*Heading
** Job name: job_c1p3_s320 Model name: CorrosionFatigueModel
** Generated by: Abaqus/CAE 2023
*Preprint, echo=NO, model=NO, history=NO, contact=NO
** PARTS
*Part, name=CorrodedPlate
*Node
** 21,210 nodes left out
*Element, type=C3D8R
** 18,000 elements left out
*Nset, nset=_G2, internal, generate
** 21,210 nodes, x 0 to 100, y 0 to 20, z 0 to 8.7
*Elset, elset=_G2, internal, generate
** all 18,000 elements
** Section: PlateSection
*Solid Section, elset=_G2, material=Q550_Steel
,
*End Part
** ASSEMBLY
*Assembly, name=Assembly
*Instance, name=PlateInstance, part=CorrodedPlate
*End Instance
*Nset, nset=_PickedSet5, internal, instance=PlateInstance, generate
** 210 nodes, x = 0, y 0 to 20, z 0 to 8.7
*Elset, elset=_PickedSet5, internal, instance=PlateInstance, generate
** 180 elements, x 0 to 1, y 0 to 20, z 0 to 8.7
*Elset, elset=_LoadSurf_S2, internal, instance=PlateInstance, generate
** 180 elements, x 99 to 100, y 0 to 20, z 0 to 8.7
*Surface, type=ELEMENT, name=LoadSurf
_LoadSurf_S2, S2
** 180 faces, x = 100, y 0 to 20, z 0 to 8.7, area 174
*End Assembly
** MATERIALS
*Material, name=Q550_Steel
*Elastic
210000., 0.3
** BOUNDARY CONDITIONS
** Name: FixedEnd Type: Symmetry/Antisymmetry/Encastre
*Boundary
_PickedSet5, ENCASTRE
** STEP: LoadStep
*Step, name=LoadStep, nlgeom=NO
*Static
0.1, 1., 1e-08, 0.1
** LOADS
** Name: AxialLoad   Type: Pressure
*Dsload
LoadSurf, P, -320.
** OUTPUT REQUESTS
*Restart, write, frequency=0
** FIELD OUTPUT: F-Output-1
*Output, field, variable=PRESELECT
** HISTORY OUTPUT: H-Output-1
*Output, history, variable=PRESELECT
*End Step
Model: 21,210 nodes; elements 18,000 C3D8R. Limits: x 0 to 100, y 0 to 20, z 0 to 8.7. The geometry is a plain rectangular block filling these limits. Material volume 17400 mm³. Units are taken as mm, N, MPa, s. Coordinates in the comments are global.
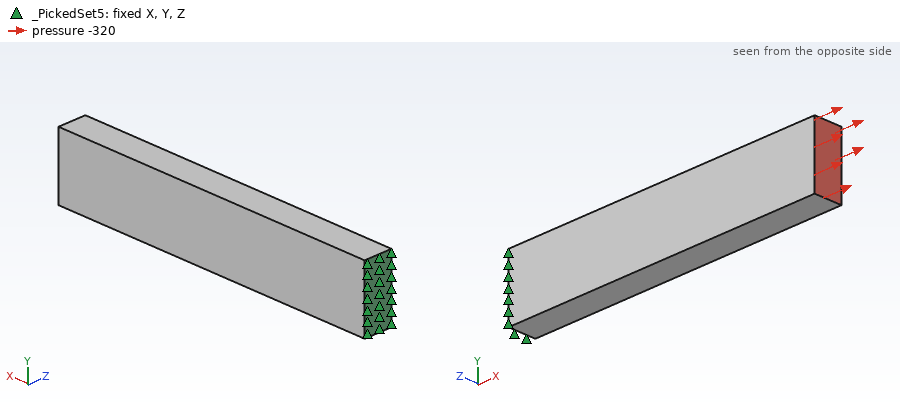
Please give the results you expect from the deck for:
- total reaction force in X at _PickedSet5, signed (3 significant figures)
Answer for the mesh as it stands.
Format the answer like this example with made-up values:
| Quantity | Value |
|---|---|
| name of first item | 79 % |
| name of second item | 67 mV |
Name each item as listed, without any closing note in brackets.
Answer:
| Quantity | Value |
|---|---|
| total reaction force in X at _PickedSet5, signed | -55700 N |
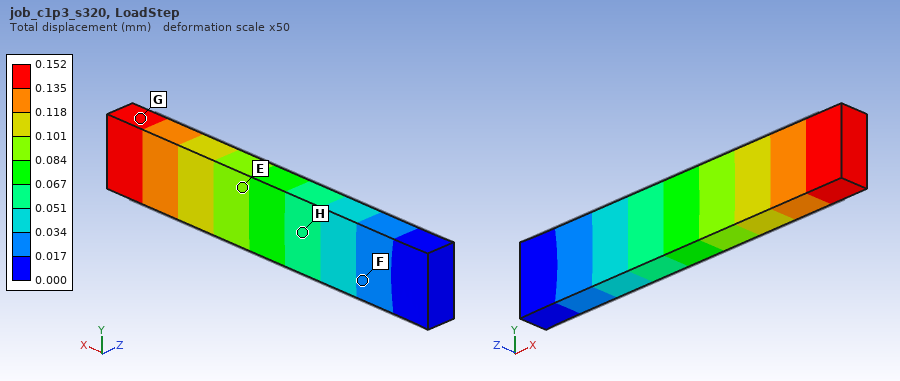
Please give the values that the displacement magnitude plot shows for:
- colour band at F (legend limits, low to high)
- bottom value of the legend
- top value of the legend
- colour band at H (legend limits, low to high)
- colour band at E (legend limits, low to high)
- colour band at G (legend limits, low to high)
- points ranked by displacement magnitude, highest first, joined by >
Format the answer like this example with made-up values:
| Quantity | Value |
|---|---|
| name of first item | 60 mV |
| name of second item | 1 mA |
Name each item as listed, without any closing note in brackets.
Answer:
| Quantity | Value |
|---|---|
| colour band at F | 0.017 to 0.034 mm |
| bottom value of the legend | 0.000 mm |
| top value of the legend | 0.152 mm |
| colour band at H | 0.051 to 0.067 mm |
| colour band at E | 0.084 to 0.101 mm |
| colour band at G | 0.135 to 0.152 mm |
| points ranked by displacement magnitude, highest first, joined by > | G > E > H > F |
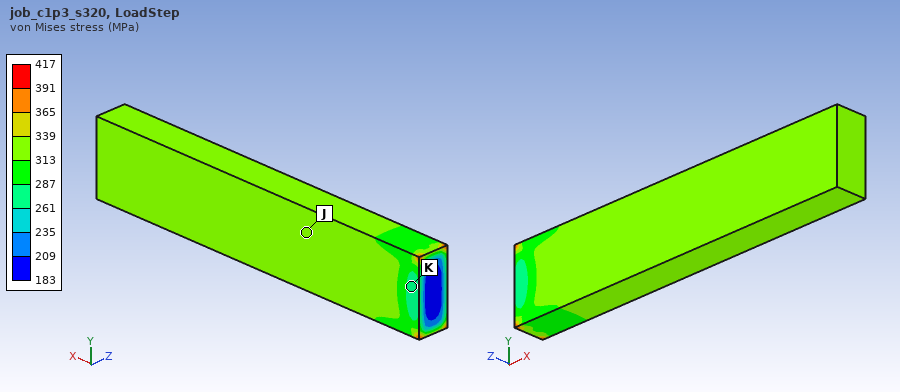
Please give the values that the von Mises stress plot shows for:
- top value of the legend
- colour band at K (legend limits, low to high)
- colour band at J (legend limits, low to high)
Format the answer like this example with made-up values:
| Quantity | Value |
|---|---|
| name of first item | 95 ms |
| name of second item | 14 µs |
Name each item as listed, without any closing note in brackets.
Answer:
| Quantity | Value |
|---|---|
| top value of the legend | 417 MPa |
| colour band at K | 261 to 287 MPa |
| colour band at J | 313 to 339 MPa |
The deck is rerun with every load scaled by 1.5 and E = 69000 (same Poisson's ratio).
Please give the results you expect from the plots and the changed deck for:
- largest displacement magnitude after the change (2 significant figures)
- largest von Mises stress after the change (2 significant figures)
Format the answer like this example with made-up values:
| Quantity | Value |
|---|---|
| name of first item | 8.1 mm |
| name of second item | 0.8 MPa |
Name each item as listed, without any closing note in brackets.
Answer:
| Quantity | Value |
|---|---|
| largest displacement magnitude after the change | 0.69 mm |
| largest von Mises stress after the change | 630 MPa |
